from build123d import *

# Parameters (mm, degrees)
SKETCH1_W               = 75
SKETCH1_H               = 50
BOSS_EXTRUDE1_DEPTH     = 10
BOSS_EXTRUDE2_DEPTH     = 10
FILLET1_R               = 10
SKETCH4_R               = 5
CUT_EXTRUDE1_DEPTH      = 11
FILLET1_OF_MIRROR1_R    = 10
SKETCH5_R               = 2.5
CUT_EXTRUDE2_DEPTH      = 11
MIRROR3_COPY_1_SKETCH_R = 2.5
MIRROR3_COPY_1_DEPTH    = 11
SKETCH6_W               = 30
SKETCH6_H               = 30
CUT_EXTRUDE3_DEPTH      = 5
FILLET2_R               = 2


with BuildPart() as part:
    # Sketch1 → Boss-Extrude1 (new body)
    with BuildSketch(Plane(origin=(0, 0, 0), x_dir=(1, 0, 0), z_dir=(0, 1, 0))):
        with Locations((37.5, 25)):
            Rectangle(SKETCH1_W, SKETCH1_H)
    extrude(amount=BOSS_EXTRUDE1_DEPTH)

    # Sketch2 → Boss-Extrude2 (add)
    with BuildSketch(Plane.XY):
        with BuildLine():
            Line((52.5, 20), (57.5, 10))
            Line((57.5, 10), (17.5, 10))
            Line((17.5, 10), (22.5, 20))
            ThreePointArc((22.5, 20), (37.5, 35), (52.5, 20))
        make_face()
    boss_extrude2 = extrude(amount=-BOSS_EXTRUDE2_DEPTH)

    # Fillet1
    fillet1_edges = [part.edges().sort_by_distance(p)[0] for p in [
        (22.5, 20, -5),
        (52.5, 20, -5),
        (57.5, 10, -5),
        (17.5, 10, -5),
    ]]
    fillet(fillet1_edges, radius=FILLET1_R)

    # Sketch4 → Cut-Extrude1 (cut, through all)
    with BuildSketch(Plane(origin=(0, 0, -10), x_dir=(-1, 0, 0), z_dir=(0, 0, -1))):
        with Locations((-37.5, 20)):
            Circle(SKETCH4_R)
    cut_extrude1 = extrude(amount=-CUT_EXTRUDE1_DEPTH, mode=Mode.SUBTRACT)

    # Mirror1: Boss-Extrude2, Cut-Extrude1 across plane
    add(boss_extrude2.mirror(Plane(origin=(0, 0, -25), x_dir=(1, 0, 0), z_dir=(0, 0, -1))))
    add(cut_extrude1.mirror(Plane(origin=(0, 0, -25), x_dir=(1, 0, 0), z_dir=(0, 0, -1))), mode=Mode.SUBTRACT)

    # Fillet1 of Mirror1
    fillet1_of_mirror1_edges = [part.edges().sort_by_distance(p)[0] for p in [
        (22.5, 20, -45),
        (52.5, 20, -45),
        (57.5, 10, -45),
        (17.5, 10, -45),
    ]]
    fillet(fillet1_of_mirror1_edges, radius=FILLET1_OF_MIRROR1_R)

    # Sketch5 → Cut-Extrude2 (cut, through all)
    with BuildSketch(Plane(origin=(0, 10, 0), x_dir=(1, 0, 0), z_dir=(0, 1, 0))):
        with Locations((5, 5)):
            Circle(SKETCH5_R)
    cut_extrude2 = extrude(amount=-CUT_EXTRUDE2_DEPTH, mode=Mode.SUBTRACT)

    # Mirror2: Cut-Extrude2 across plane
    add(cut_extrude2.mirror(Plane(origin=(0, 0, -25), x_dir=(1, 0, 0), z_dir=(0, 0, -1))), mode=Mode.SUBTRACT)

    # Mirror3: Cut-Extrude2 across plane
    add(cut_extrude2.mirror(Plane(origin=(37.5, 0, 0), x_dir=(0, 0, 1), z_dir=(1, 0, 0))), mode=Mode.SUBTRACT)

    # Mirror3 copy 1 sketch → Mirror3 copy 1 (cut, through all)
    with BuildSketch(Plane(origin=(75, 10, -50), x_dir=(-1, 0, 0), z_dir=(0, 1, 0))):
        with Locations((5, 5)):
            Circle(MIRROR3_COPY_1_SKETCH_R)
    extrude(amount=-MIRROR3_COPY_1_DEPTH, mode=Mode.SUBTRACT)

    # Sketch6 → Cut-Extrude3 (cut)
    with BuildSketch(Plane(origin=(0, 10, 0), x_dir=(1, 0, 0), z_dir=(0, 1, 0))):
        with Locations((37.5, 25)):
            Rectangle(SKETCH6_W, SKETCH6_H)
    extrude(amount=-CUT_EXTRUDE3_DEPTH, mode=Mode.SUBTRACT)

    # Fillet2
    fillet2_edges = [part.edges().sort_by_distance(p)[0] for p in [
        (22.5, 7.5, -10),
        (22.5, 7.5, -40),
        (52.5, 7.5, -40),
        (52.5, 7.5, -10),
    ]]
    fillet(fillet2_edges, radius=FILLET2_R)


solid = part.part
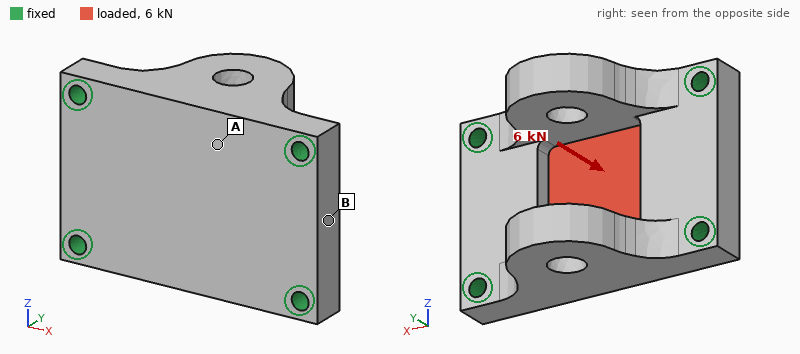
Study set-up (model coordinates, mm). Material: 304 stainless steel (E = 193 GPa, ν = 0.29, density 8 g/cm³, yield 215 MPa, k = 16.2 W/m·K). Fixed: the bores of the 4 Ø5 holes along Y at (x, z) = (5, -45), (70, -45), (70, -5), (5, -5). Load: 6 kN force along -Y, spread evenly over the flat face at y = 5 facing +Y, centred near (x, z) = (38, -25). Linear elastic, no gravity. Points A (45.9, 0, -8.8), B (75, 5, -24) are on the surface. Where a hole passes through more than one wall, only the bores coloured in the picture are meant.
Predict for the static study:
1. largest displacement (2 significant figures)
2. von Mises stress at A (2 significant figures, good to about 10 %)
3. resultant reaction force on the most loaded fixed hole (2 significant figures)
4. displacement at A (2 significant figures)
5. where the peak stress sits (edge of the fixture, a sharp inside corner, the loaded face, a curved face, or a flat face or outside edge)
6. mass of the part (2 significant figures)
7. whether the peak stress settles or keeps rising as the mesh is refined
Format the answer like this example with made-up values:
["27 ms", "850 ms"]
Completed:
["19 µm", "28 MPa", "1.5 kN", "8.3 µm", "edge of the fixture", "360 g", "keeps rising"]
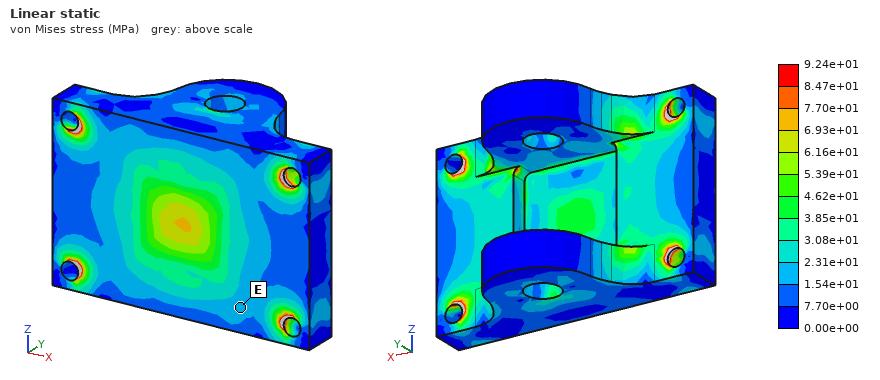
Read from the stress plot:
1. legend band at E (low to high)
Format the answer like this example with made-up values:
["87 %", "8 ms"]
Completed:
["1.54e+01 to 2.31e+01 MPa"]
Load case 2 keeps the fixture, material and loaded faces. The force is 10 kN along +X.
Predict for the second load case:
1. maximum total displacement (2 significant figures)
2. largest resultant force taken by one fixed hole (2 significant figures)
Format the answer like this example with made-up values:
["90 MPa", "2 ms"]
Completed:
["4.3 µm", "2.6 kN"]
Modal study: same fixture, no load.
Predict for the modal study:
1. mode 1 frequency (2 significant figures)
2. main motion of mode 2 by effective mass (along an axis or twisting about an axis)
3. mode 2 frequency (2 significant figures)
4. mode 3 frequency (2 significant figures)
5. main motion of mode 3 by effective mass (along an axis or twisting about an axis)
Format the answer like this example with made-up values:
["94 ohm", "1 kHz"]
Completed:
["6500 Hz", "along Z", "6900 Hz", "10 kHz", "along Y"]
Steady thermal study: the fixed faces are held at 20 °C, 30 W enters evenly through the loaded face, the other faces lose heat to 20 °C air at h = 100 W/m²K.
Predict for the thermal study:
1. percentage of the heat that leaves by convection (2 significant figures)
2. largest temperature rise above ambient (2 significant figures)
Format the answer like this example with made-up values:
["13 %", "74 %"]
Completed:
["57 %", "55 K"]
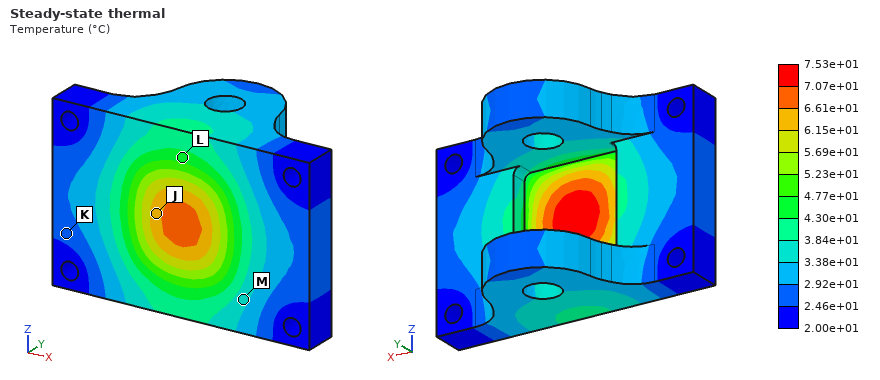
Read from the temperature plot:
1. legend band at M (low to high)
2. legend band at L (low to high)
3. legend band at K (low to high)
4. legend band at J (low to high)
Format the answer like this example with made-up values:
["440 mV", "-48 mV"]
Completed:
["3.38e+01 to 3.84e+01 °C", "4.30e+01 to 4.77e+01 °C", "2.46e+01 to 2.92e+01 °C", "6.15e+01 to 6.61e+01 °C"]
